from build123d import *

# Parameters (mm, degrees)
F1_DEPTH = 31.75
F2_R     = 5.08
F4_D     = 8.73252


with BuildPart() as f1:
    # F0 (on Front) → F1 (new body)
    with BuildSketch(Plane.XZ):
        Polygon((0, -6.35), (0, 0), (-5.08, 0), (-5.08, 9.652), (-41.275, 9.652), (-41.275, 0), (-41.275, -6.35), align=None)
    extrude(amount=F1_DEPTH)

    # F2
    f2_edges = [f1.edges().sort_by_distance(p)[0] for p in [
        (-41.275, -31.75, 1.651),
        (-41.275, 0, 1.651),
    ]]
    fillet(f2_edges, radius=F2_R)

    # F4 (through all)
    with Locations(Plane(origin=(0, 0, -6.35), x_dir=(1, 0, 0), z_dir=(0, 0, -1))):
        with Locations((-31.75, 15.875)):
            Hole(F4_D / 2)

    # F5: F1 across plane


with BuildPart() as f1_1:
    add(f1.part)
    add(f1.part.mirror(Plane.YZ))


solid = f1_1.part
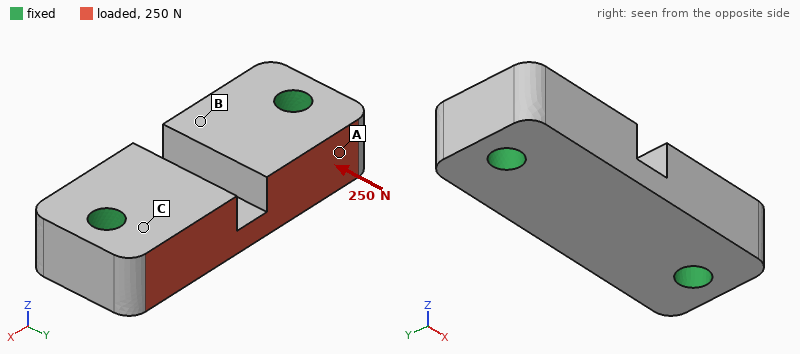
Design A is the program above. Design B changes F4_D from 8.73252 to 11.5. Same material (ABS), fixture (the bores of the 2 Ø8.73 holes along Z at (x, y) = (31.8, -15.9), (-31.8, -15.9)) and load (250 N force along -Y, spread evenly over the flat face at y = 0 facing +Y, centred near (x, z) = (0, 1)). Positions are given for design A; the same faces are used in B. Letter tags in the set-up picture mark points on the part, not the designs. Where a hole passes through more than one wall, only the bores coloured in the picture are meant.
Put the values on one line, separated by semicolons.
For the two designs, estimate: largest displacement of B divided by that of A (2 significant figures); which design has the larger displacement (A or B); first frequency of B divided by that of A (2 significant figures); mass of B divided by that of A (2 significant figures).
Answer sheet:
0.80; A; 1.1; 0.96
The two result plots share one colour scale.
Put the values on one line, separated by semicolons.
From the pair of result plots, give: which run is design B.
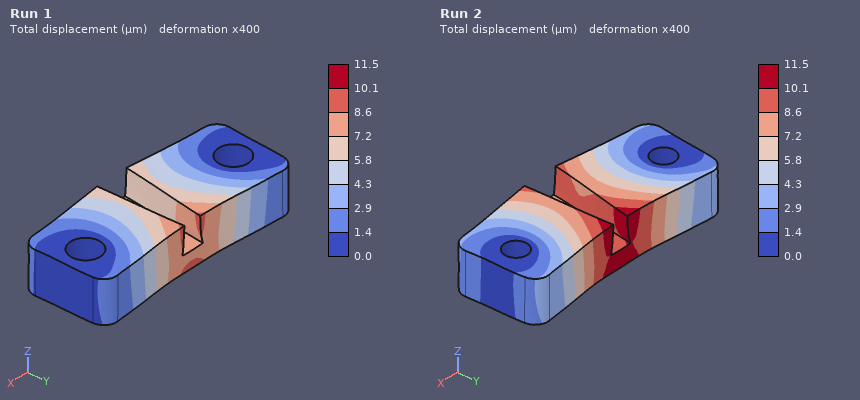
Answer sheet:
Run 1
